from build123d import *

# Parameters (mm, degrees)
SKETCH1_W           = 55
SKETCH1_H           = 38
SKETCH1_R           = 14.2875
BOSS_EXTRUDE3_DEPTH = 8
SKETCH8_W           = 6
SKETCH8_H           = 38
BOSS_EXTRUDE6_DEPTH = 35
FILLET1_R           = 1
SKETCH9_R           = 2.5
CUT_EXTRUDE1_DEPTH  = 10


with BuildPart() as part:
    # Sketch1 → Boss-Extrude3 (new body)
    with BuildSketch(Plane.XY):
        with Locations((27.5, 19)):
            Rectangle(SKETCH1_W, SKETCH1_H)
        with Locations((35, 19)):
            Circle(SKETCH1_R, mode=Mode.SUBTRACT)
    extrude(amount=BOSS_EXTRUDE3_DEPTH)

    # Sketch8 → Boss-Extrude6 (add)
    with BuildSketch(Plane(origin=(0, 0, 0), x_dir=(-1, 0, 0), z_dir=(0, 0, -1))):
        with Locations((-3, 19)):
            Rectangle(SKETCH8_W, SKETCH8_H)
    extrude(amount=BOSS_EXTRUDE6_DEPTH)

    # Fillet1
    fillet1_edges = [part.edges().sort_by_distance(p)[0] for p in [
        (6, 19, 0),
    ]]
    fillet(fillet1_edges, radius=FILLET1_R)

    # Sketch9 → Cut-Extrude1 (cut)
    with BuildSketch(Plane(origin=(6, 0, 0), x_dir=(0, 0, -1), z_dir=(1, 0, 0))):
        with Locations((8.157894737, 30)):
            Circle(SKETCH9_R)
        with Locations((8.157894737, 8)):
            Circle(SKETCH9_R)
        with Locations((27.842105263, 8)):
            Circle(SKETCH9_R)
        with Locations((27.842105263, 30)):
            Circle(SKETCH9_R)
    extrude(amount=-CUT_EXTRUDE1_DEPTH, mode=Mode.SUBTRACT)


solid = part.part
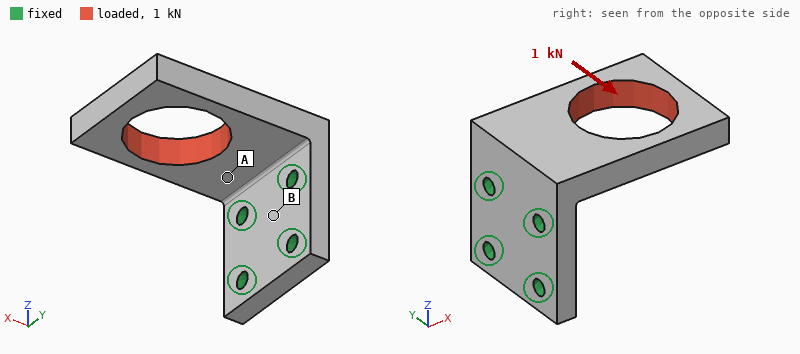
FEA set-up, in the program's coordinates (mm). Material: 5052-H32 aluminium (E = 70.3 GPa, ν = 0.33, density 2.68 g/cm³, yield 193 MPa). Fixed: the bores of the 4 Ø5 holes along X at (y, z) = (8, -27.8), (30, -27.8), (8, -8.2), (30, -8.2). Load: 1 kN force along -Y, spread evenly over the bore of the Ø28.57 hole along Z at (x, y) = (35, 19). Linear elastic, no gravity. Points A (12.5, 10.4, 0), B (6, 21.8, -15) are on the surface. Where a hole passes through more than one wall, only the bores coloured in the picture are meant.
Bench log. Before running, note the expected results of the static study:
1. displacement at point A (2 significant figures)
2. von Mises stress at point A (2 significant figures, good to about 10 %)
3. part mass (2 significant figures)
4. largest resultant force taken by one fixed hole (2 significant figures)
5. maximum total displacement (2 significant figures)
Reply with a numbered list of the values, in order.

1. 0.018 mm
2. 21 MPa
3. 51 g
4. 1.4 kN
5. 0.12 mm
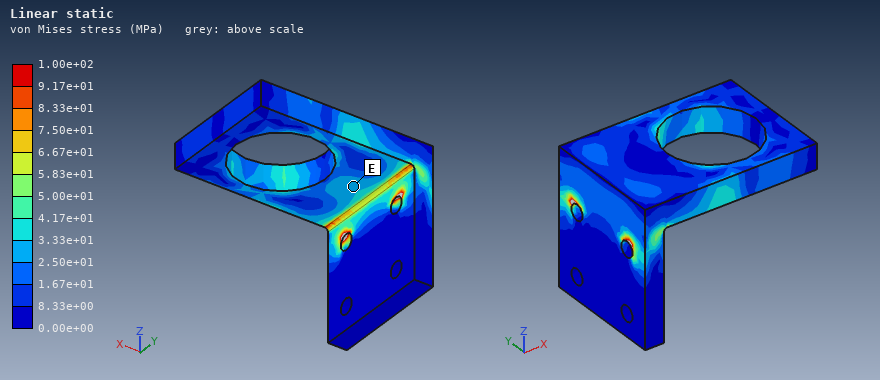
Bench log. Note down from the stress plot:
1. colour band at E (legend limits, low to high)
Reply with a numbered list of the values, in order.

1. 2.50e+01 to 3.33e+01 MPa
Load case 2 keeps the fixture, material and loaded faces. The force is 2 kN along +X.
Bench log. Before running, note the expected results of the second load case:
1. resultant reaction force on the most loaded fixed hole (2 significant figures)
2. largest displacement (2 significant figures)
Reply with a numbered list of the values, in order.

1. 1.1 kN
2. 0.16 mm
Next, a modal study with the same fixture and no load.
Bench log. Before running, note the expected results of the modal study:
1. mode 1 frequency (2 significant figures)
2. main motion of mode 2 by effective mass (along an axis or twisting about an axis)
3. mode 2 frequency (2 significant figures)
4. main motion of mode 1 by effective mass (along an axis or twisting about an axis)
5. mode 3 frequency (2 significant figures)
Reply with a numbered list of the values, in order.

1. 1700 Hz
2. along Y
3. 3700 Hz
4. along Z
5. 5100 Hz
